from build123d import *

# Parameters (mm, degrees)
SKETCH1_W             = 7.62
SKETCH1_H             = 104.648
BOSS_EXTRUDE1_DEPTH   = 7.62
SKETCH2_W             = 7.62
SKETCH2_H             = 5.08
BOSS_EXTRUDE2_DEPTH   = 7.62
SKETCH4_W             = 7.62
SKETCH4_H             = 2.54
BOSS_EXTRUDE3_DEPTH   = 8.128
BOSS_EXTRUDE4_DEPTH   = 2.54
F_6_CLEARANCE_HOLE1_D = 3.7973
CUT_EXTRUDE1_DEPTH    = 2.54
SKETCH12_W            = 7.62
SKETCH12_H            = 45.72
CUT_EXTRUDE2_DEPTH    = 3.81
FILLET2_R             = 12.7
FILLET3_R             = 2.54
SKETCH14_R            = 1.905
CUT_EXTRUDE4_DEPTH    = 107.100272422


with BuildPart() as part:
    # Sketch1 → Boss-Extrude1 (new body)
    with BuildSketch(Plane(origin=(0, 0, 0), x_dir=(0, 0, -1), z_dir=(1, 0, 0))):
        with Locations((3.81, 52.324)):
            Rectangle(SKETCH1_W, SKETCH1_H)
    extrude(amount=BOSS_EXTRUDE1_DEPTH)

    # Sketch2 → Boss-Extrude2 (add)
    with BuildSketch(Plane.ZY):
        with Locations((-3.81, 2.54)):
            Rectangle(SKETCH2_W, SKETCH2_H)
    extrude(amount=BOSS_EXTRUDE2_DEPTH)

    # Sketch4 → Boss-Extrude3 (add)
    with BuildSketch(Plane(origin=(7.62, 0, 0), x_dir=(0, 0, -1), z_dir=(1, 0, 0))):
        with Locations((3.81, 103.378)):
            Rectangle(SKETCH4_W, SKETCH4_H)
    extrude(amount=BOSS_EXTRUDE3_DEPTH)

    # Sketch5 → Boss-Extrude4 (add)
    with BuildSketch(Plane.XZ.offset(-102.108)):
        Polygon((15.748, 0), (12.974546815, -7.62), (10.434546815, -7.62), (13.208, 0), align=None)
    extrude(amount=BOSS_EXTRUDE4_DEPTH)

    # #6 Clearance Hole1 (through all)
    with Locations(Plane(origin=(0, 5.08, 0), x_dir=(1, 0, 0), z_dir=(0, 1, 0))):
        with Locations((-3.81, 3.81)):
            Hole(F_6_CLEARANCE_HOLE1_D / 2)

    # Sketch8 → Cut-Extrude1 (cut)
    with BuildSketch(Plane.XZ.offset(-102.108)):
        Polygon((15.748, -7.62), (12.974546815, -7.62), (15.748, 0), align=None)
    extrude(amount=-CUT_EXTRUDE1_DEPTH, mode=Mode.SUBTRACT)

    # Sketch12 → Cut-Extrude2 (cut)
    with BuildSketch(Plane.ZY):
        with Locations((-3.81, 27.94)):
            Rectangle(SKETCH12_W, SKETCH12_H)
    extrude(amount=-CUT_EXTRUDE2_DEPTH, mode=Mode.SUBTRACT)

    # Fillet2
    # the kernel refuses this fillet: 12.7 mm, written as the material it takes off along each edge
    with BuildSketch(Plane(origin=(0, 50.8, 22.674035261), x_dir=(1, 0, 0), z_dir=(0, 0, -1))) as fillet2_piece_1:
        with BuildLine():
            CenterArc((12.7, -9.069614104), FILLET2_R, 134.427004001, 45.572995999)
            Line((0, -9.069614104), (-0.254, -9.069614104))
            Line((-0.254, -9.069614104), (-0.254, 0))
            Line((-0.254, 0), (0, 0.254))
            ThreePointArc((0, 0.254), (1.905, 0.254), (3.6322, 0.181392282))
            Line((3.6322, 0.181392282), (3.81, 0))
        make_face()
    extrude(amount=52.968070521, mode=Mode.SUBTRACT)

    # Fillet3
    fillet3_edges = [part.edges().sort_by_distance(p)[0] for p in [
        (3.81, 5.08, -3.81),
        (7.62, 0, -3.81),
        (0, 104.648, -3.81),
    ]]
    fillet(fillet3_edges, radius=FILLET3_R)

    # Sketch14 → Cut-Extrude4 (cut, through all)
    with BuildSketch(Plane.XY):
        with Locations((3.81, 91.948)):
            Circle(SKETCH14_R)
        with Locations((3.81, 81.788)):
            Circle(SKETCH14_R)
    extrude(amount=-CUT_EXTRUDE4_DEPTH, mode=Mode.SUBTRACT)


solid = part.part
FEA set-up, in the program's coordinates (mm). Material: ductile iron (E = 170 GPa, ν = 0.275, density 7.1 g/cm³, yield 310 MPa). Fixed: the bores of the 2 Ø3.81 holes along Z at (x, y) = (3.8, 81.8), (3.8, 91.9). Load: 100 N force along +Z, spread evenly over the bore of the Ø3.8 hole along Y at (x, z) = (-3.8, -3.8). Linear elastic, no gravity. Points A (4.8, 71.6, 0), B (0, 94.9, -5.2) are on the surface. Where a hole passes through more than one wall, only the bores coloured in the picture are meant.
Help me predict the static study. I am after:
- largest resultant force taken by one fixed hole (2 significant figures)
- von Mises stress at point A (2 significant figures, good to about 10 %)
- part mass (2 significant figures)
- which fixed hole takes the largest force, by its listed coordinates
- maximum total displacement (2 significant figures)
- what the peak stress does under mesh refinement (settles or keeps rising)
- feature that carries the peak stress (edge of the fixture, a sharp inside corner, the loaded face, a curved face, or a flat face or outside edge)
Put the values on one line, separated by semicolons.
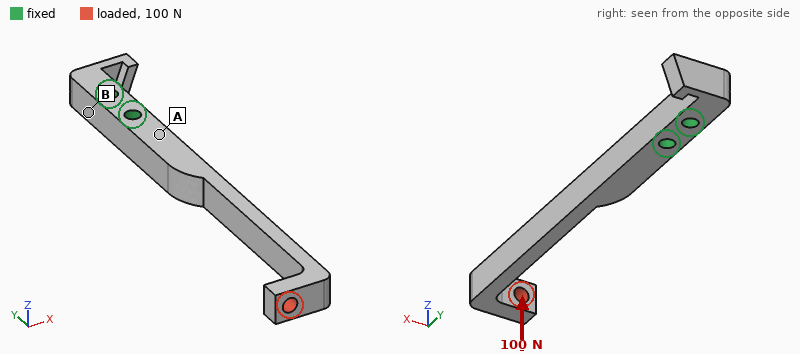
140 N; 95 MPa; 35 g; (3.8, 81.8); 0.57 mm; keeps rising; edge of the fixture
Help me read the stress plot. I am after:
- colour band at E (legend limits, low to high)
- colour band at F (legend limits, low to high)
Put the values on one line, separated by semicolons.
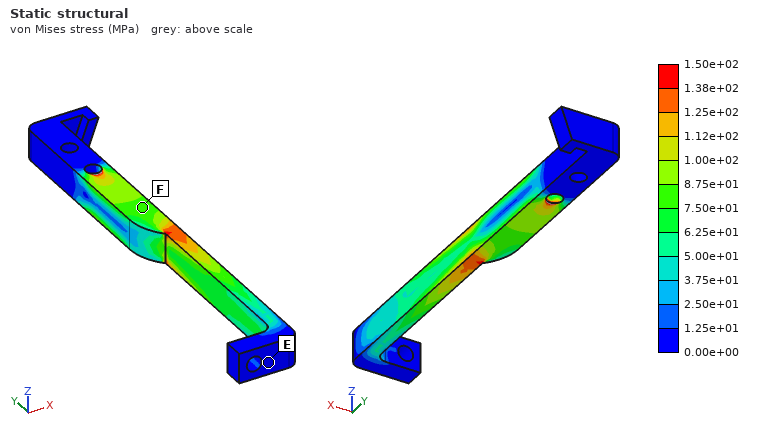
0.00e+00 to 1.25e+01 MPa; 7.50e+01 to 8.75e+01 MPa
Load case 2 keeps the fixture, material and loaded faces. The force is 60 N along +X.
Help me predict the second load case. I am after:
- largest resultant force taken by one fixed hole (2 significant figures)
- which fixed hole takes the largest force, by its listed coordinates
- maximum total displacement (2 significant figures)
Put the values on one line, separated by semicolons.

150 N; (3.8, 81.8); 0.66 mm
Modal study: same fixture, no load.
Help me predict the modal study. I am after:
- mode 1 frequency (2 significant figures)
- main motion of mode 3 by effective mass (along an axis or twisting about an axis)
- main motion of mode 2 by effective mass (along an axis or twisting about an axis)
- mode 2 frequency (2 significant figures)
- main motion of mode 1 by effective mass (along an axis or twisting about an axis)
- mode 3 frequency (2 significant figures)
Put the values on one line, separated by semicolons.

640 Hz; along X; along Z; 910 Hz; along X; 3200 Hz
